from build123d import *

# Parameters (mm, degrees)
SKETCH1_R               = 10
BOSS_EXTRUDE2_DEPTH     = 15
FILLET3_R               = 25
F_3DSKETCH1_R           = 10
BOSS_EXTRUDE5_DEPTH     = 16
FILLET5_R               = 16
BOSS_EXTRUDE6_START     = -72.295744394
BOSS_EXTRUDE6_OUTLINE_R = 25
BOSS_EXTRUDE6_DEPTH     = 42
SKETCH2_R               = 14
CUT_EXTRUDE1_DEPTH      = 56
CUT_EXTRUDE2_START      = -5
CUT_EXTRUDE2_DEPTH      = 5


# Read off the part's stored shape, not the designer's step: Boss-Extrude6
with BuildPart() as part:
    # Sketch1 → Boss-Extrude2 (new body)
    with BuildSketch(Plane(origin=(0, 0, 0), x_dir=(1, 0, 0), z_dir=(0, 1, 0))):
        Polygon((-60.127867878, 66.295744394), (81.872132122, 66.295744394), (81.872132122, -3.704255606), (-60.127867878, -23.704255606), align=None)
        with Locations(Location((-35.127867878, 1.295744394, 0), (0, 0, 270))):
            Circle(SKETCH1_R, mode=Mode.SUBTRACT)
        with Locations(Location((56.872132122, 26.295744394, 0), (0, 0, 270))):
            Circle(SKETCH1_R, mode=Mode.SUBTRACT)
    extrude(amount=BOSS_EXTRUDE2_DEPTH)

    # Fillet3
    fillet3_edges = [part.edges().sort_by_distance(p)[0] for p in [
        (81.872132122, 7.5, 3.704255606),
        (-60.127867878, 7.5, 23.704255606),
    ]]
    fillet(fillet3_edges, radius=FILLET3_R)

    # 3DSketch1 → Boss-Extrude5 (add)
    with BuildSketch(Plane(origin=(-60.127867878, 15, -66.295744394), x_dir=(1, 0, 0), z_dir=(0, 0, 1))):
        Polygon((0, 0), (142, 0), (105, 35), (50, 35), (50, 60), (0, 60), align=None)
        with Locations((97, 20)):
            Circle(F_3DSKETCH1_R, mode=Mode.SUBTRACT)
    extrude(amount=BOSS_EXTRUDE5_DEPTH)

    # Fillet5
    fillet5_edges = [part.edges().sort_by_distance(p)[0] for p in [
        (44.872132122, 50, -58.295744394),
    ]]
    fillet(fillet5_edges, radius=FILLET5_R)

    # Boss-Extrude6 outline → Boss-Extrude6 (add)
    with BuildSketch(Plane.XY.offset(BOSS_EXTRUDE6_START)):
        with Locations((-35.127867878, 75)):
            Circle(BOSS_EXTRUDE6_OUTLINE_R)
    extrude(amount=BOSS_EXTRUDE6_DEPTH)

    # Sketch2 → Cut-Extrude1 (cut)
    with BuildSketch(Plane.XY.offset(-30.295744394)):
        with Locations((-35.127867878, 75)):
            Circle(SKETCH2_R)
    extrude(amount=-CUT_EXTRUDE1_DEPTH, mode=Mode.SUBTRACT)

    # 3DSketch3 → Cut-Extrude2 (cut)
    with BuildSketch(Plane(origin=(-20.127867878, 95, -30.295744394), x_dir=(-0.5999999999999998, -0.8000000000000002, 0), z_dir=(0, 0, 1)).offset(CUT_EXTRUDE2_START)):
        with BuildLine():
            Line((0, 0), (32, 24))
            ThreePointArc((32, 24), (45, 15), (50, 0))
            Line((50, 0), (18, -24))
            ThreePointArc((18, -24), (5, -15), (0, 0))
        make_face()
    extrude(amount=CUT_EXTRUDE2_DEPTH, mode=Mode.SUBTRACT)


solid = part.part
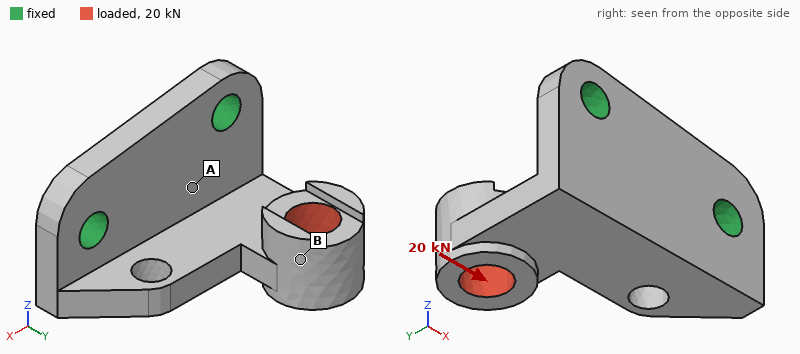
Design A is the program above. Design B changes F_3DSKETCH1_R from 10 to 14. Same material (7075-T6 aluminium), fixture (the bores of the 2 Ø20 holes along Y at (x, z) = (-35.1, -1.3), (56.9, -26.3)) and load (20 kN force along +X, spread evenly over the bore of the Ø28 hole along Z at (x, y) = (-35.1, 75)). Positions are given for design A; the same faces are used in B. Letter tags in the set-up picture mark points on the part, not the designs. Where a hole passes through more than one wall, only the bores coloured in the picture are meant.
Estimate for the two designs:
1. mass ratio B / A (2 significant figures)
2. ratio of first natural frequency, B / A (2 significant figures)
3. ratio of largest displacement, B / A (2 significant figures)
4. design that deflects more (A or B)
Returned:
0.98
0.99
1.1
B
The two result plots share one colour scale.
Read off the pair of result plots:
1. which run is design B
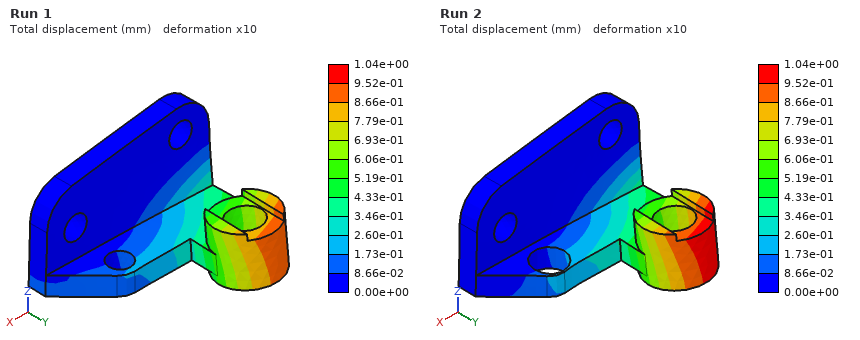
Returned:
Run 2
